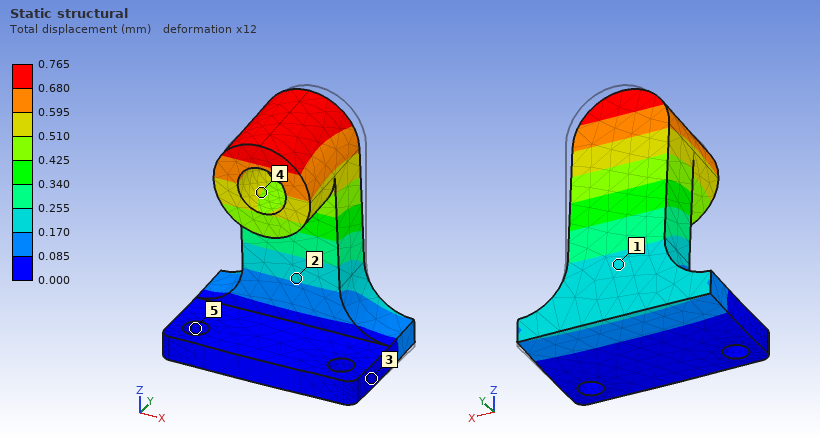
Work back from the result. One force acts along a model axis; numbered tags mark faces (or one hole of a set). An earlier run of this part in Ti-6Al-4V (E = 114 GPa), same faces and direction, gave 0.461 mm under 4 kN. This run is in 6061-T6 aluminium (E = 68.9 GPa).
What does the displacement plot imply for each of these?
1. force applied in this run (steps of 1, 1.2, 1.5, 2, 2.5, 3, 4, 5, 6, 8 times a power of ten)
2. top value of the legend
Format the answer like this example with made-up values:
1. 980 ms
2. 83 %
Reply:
1. 4 kN
2. 0.765 mm
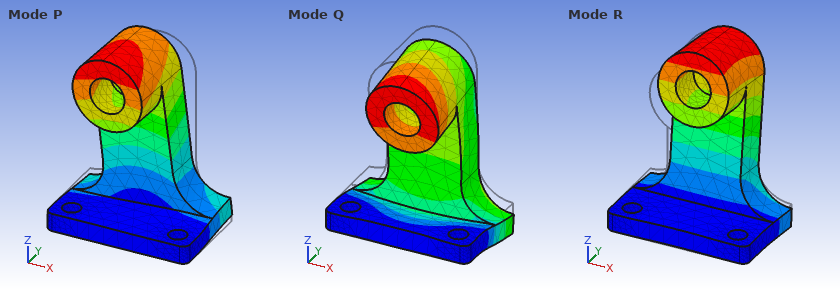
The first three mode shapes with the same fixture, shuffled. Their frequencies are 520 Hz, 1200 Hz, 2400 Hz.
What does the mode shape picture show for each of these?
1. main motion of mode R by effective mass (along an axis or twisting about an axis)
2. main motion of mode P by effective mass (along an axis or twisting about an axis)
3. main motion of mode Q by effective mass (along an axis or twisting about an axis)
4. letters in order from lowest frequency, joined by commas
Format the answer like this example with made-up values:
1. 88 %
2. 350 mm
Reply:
1. along Y
2. along X
3. along Z
4. R, P, Q
